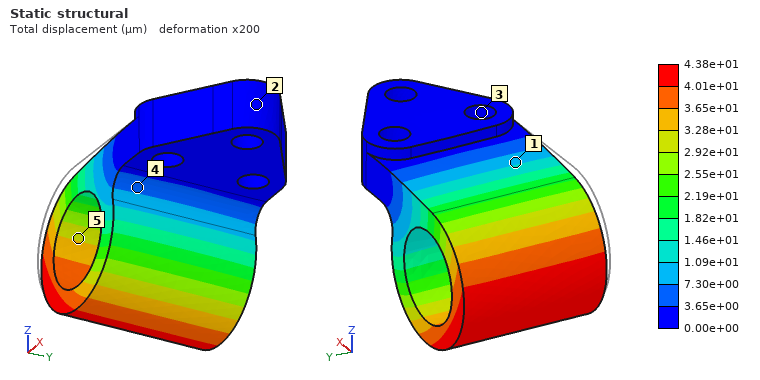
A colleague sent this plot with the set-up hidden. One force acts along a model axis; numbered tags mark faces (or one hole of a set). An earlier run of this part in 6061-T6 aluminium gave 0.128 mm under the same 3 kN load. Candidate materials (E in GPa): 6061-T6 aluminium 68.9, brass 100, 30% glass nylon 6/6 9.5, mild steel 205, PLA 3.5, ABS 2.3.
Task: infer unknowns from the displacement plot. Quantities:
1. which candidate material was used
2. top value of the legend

mild steel
4.38e+01 µm
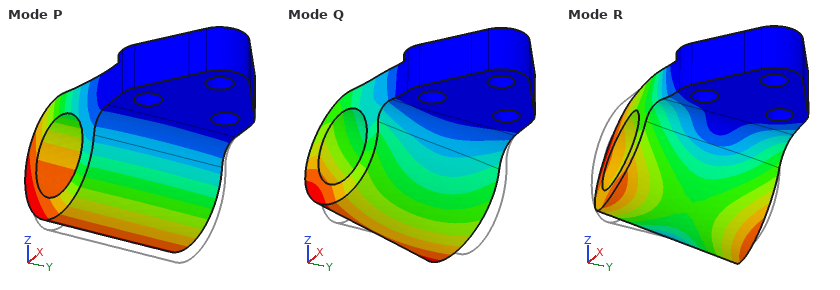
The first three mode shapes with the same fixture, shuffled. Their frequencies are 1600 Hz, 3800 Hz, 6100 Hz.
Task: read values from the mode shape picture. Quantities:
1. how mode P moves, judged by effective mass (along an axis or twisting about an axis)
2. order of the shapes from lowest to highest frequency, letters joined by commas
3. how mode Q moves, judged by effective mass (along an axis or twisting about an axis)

along Z
P, Q, R
along Y
